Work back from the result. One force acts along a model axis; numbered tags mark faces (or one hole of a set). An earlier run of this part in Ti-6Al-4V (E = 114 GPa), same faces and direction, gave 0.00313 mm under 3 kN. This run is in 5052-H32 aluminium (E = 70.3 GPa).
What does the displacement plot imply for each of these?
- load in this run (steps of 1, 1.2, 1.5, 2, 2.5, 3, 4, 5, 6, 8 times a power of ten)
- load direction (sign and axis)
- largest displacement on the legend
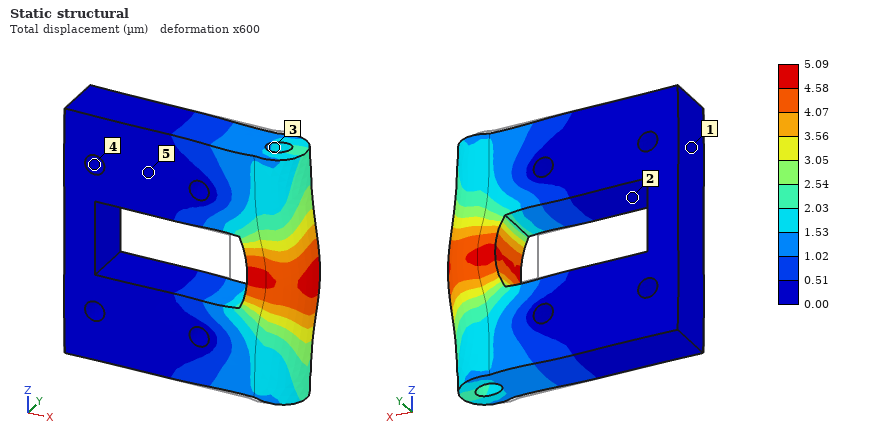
3 kN
+X
5.09 µm
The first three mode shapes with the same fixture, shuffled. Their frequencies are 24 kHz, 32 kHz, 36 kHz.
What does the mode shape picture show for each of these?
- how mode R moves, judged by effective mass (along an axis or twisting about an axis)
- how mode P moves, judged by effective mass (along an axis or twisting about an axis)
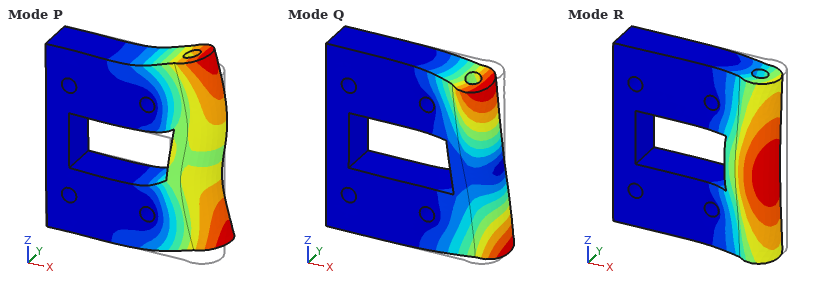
along Y
along Z
